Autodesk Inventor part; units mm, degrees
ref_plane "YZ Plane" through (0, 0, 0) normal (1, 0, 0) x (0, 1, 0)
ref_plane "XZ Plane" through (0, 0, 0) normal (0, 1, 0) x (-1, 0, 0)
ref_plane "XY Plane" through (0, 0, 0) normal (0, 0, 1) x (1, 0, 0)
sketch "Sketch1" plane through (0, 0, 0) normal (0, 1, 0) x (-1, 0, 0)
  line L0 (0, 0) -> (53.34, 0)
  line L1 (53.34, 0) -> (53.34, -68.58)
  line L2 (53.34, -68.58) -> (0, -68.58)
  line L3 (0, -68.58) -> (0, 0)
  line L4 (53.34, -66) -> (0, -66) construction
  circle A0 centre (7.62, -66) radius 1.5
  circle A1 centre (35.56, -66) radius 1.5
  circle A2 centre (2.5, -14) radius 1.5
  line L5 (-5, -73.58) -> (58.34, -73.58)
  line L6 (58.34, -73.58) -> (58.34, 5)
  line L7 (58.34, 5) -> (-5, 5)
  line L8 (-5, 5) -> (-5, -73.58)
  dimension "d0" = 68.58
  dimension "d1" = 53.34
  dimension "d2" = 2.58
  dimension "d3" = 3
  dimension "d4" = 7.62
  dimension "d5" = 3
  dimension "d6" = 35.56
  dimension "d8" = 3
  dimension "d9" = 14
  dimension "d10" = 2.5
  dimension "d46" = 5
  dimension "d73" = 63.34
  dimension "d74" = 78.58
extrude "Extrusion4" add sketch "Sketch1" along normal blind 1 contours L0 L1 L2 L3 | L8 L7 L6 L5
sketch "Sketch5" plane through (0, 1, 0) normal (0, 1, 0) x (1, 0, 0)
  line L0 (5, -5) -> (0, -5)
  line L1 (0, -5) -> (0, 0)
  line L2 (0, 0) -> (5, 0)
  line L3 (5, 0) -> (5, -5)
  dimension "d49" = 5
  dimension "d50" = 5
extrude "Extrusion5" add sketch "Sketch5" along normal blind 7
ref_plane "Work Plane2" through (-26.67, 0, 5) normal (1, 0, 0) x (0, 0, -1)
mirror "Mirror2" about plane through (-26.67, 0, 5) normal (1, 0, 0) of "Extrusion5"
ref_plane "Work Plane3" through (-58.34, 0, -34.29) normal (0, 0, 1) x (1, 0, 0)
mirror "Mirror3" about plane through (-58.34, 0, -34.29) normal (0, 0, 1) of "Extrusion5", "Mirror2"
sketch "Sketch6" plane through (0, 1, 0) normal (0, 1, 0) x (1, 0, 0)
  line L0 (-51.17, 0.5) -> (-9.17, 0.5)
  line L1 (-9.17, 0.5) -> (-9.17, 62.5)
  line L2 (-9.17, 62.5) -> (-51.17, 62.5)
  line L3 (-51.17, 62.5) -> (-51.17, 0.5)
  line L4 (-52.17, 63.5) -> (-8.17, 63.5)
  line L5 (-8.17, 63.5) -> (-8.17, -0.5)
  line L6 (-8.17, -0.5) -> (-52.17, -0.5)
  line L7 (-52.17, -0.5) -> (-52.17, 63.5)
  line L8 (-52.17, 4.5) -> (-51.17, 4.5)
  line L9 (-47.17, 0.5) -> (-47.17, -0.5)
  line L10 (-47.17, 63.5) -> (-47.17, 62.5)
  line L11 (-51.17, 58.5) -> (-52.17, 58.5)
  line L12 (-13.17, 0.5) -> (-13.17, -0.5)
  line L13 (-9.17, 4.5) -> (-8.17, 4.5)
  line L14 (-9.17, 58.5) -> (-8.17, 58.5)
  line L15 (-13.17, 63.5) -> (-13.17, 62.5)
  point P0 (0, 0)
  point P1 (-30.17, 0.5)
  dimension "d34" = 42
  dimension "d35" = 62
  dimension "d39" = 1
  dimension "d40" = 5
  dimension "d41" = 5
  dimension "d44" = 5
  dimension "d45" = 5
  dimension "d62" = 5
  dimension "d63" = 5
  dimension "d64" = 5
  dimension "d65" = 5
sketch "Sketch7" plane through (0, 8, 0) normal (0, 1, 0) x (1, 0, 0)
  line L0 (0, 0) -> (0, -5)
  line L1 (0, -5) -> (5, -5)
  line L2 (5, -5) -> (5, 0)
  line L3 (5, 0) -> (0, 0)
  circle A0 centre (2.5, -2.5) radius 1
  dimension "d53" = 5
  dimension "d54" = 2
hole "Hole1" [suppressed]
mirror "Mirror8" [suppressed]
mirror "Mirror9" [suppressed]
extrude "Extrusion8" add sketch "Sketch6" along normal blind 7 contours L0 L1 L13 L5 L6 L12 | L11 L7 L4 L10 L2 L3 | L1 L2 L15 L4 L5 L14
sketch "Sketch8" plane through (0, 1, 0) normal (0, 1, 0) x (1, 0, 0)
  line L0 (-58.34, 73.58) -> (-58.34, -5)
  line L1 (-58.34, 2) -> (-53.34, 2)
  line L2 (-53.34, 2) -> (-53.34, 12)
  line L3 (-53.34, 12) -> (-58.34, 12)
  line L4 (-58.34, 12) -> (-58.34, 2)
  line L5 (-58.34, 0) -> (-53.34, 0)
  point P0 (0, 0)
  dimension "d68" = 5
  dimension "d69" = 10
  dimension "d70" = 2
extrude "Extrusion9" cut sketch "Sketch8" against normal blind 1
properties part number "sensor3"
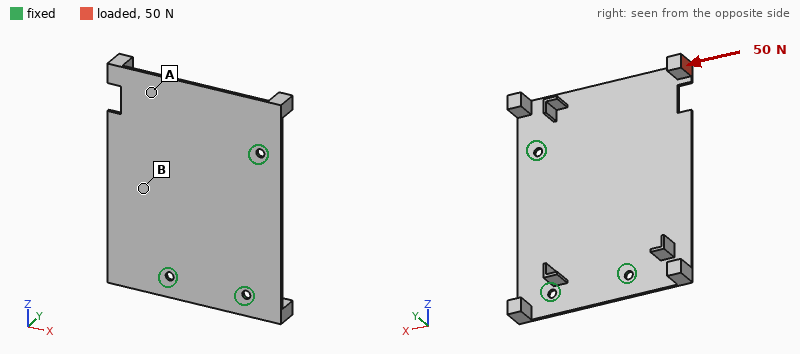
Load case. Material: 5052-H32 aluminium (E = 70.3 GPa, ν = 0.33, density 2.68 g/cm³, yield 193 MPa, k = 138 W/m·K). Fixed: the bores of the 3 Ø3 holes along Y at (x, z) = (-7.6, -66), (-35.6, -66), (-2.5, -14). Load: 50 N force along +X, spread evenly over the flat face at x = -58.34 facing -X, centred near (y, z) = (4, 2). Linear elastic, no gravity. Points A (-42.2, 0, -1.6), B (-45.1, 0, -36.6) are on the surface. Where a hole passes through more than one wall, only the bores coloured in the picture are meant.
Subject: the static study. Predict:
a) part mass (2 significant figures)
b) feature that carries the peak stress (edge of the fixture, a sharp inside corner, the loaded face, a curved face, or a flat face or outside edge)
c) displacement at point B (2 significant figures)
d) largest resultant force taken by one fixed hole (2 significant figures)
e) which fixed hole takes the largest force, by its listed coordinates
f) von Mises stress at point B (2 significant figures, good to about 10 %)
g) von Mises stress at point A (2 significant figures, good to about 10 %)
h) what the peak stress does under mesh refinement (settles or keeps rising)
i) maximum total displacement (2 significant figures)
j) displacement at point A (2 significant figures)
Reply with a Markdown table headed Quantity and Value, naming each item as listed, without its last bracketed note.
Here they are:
| Quantity | Value |
|---|---|
| part mass | 16 g |
| feature that carries the peak stress | a sharp inside corner |
| displacement at point B | 0.15 mm |
| largest resultant force taken by one fixed hole | 56 N |
| which fixed hole takes the largest force, by its listed coordinates | (-2.5, -14) |
| von Mises stress at point B | 13 MPa |
| von Mises stress at point A | 33 MPa |
| what the peak stress does under mesh refinement | keeps rising |
| maximum total displacement | 0.93 mm |
| displacement at point A | 0.30 mm |
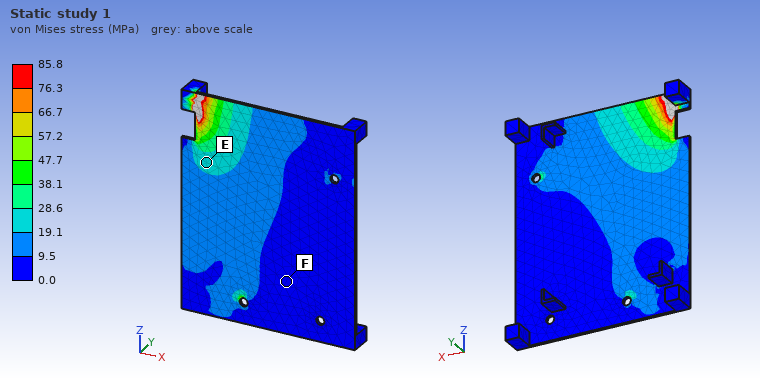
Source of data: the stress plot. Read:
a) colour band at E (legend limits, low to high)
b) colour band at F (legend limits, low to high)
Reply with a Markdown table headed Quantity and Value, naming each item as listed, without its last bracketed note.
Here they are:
| Quantity | Value |
|---|---|
| colour band at E | 19.1 to 28.6 MPa |
| colour band at F | 0.0 to 9.5 MPa |
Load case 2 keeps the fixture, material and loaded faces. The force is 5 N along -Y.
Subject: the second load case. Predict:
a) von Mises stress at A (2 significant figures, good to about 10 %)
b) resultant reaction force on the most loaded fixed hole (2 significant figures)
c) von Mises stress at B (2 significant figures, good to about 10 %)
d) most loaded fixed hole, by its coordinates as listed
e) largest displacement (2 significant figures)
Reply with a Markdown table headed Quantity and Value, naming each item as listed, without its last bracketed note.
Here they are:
| Quantity | Value |
|---|---|
| von Mises stress at A | 21 MPa |
| resultant reaction force on the most loaded fixed hole | 4.6 N |
| von Mises stress at B | 14 MPa |
| most loaded fixed hole, by its coordinates as listed | (-2.5, -14) |
| largest displacement | 1.0 mm |
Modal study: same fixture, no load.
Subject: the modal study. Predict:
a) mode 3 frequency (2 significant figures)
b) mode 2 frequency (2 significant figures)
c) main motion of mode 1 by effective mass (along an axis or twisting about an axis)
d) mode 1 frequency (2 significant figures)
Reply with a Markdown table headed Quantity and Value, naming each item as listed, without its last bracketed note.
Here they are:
| Quantity | Value |
|---|---|
| mode 3 frequency | 1200 Hz |
| mode 2 frequency | 920 Hz |
| main motion of mode 1 by effective mass | along Y |
| mode 1 frequency | 330 Hz |
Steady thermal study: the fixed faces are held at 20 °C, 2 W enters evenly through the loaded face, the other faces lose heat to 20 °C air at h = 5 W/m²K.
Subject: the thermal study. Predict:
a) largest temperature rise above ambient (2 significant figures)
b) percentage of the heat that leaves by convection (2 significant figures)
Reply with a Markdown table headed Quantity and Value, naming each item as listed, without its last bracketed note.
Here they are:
| Quantity | Value |
|---|---|
| largest temperature rise above ambient | 32 K |
| percentage of the heat that leaves by convection | 12 % |
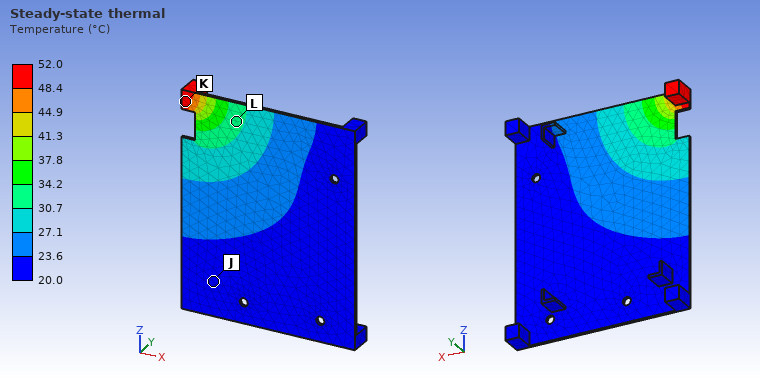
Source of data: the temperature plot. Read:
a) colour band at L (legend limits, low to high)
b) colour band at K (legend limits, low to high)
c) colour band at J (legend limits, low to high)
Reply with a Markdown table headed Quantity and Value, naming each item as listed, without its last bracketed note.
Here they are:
| Quantity | Value |
|---|---|
| colour band at L | 30.7 to 34.2 °C |
| colour band at K | 48.4 to 52.0 °C |
| colour band at J | 20.0 to 23.6 °C |
